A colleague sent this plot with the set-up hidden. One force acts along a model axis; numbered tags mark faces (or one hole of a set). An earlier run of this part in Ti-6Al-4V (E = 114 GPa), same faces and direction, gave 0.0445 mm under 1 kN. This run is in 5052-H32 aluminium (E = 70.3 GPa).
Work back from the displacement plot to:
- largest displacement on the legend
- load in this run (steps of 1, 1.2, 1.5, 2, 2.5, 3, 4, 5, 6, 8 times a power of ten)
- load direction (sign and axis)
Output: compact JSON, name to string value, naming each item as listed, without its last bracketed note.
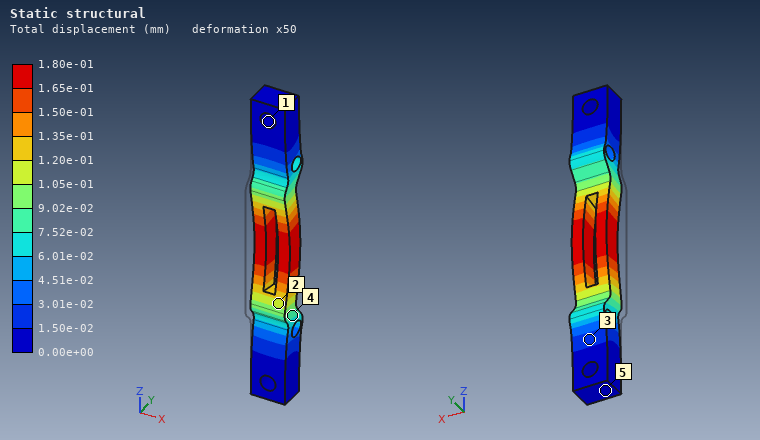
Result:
{"largest displacement on the legend": "1.80e-01 mm", "load in this run": "2.5 kN", "load direction": "+Y"}
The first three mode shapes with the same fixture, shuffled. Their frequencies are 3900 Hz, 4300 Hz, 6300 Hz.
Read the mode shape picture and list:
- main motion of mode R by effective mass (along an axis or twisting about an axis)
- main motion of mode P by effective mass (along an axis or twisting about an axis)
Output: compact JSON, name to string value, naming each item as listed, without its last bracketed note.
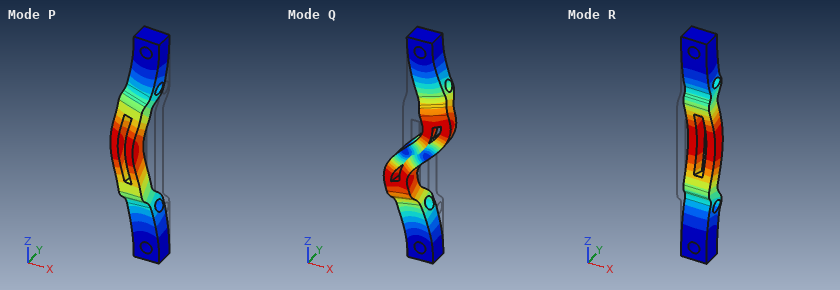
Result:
{"main motion of mode R by effective mass": "along Y", "main motion of mode P by effective mass": "along X"}
